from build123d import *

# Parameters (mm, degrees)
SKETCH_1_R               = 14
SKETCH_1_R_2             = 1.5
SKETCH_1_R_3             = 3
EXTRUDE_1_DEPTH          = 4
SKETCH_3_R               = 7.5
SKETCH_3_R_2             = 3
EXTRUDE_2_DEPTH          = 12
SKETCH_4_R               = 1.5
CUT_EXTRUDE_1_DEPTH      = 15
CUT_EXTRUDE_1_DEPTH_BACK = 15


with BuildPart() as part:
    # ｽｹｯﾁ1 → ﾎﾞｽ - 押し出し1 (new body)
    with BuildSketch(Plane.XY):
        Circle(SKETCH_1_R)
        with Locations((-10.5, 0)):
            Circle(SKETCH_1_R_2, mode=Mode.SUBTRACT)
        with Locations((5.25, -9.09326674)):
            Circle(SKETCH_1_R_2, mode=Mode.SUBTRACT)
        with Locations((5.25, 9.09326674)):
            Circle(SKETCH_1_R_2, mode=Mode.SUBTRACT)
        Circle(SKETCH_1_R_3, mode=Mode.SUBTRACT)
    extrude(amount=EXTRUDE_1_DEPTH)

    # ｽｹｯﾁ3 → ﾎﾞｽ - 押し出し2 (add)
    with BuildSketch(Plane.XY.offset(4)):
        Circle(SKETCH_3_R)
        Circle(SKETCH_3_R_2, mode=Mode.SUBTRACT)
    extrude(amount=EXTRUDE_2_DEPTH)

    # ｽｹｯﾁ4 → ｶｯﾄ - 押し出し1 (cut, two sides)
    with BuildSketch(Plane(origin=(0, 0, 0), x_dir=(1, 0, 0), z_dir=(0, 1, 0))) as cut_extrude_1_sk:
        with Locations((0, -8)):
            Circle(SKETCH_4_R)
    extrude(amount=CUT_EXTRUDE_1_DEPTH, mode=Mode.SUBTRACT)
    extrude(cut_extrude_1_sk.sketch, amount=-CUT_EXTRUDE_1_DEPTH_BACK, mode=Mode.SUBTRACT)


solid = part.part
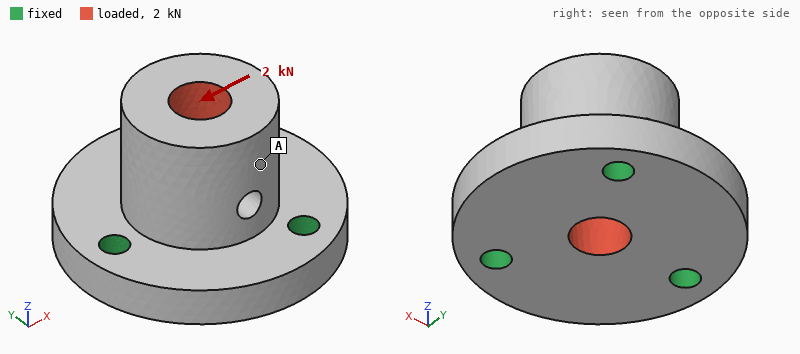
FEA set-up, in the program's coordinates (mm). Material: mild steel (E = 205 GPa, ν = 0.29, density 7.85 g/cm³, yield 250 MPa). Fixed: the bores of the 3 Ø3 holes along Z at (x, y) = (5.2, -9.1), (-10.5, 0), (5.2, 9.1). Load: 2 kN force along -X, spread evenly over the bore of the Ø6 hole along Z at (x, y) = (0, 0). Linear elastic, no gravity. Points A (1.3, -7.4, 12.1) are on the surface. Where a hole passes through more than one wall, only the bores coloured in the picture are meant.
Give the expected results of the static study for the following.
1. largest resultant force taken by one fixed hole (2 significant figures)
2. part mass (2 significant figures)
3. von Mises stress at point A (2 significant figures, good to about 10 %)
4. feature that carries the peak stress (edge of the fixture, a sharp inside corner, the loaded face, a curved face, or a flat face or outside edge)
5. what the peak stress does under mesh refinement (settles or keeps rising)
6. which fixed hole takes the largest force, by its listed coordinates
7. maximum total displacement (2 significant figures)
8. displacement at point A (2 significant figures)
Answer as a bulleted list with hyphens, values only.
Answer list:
- 1.1 kN
- 31 g
- 11 MPa
- edge of the fixture
- keeps rising
- (-10.5, 0)
- 5.9 µm
- 4.0 µm
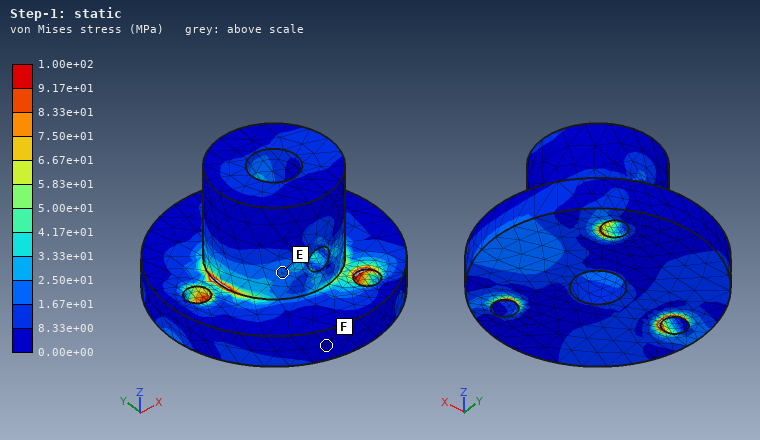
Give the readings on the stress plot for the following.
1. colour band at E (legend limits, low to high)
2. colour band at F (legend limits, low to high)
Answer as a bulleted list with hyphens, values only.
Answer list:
- 1.67e+01 to 2.50e+01 MPa
- 0.00e+00 to 8.33e+00 MPa
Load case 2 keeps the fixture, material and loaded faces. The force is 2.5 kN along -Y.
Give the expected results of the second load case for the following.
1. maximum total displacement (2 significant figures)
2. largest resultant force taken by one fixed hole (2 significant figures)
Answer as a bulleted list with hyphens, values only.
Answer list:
- 7.3 µm
- 1.2 kN
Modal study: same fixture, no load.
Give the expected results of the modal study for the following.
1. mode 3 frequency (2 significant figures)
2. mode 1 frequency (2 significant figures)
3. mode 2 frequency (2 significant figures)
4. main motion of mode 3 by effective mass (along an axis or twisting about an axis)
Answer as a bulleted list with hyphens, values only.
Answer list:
- 35 kHz
- 24 kHz
- 25 kHz
- along Z
